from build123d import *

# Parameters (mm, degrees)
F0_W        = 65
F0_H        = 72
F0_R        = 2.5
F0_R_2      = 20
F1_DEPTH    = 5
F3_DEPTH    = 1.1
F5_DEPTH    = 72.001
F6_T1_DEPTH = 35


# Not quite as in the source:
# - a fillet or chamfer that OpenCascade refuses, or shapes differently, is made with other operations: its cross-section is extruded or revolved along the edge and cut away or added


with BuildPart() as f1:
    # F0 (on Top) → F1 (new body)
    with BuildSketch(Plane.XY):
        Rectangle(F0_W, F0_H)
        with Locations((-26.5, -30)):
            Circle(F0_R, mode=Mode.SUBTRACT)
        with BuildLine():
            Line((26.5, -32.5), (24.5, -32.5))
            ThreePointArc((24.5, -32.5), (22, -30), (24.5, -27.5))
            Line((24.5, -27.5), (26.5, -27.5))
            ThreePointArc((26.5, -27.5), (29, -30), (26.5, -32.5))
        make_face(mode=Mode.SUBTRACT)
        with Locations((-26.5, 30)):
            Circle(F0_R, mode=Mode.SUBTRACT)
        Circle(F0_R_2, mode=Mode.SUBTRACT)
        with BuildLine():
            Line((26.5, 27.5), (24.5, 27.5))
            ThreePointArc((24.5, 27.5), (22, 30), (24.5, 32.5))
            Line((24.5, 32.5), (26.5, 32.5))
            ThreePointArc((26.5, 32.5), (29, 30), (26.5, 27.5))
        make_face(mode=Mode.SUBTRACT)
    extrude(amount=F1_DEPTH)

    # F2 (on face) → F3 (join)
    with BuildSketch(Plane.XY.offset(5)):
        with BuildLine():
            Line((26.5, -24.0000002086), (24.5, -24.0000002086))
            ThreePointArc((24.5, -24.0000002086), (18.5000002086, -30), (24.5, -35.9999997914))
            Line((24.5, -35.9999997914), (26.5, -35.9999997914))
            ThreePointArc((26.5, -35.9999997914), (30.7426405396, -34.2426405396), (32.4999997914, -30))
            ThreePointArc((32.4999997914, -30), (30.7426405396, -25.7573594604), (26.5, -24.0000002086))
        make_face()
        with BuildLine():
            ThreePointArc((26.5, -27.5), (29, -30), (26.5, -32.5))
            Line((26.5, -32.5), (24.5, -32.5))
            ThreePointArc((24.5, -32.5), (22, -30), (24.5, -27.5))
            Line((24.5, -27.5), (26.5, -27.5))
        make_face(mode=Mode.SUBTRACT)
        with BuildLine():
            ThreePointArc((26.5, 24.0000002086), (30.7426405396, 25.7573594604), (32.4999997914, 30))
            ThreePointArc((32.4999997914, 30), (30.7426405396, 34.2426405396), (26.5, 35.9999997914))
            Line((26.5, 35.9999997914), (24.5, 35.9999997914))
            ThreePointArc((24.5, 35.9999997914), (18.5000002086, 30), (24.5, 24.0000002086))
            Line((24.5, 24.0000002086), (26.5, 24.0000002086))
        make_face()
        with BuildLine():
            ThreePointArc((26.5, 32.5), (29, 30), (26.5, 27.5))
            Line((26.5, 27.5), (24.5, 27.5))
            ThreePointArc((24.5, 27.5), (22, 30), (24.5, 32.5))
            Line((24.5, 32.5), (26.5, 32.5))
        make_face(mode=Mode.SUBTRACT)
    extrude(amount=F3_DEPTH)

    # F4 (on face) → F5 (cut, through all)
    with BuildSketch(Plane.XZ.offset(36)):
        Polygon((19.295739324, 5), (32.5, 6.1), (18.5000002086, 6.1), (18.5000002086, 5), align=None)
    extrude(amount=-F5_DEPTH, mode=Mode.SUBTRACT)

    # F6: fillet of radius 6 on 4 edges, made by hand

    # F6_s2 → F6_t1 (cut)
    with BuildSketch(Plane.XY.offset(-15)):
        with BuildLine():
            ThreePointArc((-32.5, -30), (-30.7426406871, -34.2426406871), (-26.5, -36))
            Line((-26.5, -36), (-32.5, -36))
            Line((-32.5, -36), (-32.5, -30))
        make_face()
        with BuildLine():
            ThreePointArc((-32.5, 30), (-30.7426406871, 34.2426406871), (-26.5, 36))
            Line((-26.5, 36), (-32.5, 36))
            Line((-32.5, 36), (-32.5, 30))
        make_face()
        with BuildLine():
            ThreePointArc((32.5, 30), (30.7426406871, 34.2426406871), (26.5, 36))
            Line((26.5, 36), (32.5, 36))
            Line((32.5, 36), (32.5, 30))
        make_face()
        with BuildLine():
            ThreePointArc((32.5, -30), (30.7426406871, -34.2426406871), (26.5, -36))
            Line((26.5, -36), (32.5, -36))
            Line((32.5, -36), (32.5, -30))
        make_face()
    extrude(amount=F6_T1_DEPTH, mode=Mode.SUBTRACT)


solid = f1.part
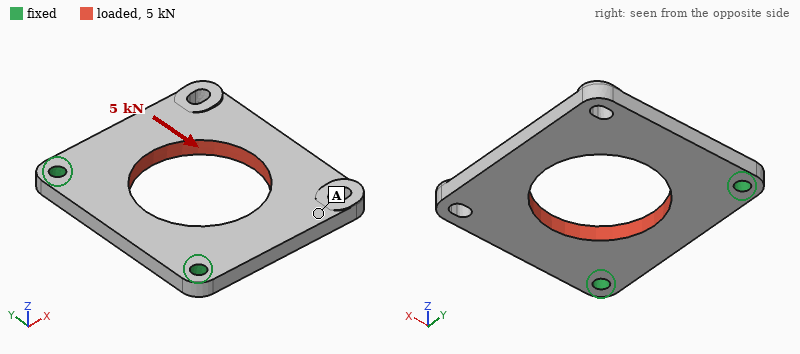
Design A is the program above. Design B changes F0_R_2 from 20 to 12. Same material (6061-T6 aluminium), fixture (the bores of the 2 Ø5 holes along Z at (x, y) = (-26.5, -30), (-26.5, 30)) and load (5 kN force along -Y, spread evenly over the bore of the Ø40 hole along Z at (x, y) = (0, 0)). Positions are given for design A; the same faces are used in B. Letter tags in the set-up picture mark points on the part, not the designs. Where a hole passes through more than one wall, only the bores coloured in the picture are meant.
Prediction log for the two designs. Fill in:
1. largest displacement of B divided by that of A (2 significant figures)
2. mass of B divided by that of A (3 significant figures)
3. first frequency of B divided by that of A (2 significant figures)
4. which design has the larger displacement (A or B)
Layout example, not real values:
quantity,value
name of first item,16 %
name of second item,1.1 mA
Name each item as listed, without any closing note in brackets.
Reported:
quantity,value
largest displacement of B divided by that of A,0.40
mass of B divided by that of A,1.24
first frequency of B divided by that of A,1.0
which design has the larger displacement,A
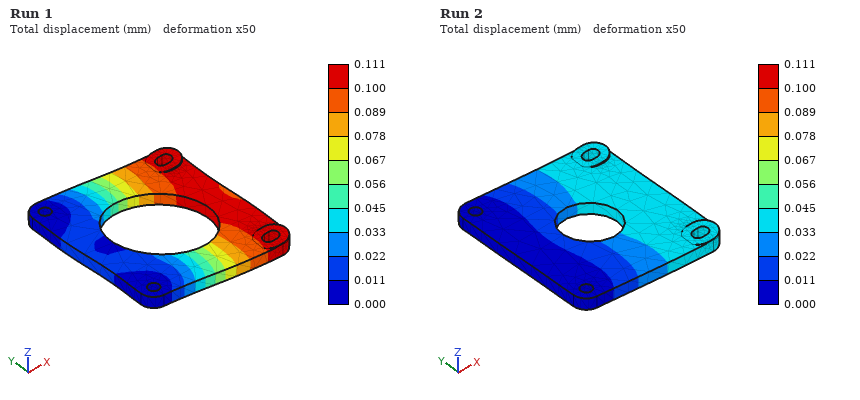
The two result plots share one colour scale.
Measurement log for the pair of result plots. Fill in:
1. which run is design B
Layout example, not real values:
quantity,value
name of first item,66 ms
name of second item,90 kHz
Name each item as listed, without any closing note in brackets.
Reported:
quantity,value
which run is design B,Run 2
